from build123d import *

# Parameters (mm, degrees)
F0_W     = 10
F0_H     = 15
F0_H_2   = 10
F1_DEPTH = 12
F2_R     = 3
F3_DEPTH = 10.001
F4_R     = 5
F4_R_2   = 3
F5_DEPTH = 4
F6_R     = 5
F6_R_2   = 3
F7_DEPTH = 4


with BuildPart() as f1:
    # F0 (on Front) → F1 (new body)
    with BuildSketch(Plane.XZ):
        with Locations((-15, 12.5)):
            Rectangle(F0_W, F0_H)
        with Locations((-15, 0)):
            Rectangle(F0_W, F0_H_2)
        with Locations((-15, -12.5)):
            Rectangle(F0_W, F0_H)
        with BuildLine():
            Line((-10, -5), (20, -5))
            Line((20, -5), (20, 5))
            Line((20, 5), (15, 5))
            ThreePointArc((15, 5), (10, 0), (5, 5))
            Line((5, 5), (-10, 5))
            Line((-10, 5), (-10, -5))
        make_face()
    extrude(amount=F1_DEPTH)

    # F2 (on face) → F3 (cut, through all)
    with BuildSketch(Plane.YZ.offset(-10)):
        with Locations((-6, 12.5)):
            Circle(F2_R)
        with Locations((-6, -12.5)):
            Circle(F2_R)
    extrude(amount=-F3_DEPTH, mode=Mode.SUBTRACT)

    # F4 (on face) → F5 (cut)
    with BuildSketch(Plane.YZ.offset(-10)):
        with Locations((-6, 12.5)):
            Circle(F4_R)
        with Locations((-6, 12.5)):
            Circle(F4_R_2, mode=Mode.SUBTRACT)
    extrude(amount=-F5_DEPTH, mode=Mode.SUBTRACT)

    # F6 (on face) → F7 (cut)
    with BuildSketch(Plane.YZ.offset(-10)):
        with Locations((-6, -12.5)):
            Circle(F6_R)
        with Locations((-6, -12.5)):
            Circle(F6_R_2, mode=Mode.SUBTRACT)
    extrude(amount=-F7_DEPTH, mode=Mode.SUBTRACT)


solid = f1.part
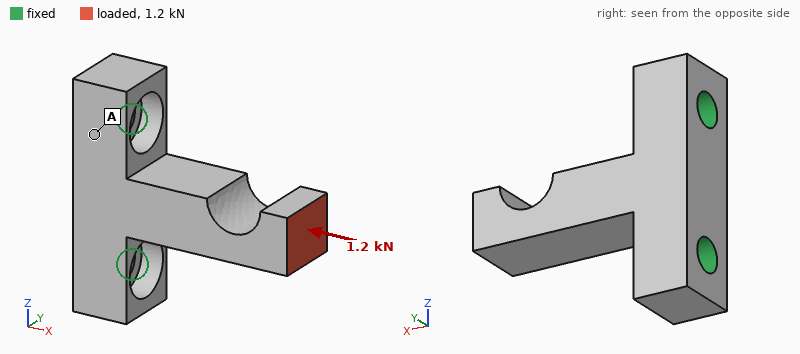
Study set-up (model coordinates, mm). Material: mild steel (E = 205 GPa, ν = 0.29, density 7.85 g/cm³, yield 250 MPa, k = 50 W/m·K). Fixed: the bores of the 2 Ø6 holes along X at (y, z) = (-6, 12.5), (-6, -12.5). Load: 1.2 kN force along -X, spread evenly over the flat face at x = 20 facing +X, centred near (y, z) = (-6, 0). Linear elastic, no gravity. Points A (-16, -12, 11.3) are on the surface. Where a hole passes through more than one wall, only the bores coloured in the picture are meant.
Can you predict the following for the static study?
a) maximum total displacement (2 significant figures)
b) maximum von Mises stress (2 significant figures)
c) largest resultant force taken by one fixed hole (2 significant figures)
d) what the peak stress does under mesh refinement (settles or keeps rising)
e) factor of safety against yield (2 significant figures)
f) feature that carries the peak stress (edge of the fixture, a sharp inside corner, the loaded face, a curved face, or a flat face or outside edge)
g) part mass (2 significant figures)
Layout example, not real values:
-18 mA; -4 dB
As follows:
13 µm; 92 MPa; 660 N; settles; 2.7; a curved face; 55 g
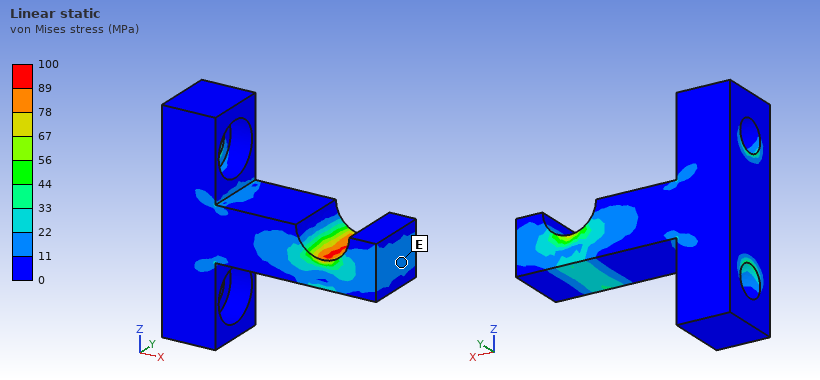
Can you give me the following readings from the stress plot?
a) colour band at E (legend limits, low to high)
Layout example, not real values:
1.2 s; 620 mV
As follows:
11 to 22 MPa
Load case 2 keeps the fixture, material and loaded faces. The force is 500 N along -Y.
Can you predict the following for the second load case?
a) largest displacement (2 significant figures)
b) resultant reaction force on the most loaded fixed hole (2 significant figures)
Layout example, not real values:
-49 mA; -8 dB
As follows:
54 µm; 250 N
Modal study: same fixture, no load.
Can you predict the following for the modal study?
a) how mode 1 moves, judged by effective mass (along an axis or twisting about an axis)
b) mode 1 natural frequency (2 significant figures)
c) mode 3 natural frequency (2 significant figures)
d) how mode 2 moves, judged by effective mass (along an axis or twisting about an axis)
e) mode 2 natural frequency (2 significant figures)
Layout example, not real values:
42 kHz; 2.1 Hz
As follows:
along Y; 5500 Hz; 20 kHz; along Z; 6800 Hz
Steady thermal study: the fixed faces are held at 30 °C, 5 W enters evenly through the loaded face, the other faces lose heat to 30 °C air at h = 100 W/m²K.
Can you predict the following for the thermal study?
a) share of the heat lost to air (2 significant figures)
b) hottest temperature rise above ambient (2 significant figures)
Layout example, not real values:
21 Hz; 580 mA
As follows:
42 %; 30 K
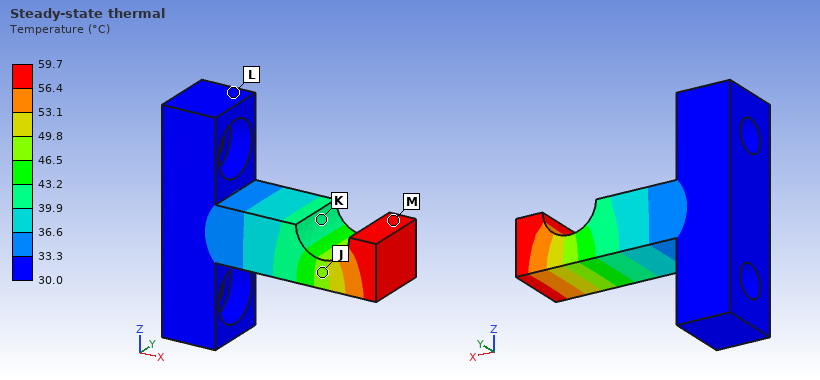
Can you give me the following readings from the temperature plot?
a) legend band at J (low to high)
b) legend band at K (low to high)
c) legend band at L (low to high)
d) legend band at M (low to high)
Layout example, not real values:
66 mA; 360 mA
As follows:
46.5 to 49.8 °C; 39.9 to 43.2 °C; 30.0 to 33.3 °C; 56.4 to 59.7 °C
